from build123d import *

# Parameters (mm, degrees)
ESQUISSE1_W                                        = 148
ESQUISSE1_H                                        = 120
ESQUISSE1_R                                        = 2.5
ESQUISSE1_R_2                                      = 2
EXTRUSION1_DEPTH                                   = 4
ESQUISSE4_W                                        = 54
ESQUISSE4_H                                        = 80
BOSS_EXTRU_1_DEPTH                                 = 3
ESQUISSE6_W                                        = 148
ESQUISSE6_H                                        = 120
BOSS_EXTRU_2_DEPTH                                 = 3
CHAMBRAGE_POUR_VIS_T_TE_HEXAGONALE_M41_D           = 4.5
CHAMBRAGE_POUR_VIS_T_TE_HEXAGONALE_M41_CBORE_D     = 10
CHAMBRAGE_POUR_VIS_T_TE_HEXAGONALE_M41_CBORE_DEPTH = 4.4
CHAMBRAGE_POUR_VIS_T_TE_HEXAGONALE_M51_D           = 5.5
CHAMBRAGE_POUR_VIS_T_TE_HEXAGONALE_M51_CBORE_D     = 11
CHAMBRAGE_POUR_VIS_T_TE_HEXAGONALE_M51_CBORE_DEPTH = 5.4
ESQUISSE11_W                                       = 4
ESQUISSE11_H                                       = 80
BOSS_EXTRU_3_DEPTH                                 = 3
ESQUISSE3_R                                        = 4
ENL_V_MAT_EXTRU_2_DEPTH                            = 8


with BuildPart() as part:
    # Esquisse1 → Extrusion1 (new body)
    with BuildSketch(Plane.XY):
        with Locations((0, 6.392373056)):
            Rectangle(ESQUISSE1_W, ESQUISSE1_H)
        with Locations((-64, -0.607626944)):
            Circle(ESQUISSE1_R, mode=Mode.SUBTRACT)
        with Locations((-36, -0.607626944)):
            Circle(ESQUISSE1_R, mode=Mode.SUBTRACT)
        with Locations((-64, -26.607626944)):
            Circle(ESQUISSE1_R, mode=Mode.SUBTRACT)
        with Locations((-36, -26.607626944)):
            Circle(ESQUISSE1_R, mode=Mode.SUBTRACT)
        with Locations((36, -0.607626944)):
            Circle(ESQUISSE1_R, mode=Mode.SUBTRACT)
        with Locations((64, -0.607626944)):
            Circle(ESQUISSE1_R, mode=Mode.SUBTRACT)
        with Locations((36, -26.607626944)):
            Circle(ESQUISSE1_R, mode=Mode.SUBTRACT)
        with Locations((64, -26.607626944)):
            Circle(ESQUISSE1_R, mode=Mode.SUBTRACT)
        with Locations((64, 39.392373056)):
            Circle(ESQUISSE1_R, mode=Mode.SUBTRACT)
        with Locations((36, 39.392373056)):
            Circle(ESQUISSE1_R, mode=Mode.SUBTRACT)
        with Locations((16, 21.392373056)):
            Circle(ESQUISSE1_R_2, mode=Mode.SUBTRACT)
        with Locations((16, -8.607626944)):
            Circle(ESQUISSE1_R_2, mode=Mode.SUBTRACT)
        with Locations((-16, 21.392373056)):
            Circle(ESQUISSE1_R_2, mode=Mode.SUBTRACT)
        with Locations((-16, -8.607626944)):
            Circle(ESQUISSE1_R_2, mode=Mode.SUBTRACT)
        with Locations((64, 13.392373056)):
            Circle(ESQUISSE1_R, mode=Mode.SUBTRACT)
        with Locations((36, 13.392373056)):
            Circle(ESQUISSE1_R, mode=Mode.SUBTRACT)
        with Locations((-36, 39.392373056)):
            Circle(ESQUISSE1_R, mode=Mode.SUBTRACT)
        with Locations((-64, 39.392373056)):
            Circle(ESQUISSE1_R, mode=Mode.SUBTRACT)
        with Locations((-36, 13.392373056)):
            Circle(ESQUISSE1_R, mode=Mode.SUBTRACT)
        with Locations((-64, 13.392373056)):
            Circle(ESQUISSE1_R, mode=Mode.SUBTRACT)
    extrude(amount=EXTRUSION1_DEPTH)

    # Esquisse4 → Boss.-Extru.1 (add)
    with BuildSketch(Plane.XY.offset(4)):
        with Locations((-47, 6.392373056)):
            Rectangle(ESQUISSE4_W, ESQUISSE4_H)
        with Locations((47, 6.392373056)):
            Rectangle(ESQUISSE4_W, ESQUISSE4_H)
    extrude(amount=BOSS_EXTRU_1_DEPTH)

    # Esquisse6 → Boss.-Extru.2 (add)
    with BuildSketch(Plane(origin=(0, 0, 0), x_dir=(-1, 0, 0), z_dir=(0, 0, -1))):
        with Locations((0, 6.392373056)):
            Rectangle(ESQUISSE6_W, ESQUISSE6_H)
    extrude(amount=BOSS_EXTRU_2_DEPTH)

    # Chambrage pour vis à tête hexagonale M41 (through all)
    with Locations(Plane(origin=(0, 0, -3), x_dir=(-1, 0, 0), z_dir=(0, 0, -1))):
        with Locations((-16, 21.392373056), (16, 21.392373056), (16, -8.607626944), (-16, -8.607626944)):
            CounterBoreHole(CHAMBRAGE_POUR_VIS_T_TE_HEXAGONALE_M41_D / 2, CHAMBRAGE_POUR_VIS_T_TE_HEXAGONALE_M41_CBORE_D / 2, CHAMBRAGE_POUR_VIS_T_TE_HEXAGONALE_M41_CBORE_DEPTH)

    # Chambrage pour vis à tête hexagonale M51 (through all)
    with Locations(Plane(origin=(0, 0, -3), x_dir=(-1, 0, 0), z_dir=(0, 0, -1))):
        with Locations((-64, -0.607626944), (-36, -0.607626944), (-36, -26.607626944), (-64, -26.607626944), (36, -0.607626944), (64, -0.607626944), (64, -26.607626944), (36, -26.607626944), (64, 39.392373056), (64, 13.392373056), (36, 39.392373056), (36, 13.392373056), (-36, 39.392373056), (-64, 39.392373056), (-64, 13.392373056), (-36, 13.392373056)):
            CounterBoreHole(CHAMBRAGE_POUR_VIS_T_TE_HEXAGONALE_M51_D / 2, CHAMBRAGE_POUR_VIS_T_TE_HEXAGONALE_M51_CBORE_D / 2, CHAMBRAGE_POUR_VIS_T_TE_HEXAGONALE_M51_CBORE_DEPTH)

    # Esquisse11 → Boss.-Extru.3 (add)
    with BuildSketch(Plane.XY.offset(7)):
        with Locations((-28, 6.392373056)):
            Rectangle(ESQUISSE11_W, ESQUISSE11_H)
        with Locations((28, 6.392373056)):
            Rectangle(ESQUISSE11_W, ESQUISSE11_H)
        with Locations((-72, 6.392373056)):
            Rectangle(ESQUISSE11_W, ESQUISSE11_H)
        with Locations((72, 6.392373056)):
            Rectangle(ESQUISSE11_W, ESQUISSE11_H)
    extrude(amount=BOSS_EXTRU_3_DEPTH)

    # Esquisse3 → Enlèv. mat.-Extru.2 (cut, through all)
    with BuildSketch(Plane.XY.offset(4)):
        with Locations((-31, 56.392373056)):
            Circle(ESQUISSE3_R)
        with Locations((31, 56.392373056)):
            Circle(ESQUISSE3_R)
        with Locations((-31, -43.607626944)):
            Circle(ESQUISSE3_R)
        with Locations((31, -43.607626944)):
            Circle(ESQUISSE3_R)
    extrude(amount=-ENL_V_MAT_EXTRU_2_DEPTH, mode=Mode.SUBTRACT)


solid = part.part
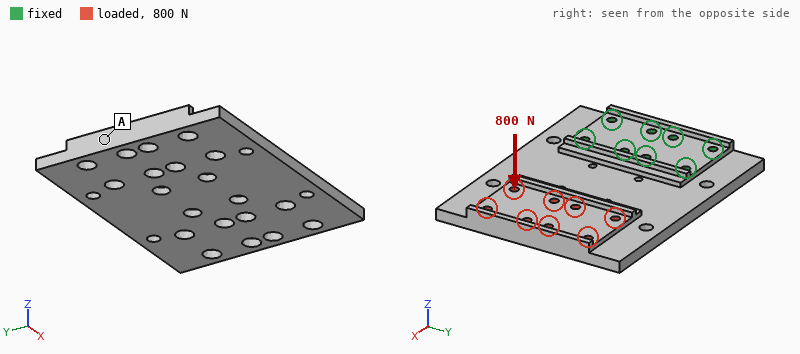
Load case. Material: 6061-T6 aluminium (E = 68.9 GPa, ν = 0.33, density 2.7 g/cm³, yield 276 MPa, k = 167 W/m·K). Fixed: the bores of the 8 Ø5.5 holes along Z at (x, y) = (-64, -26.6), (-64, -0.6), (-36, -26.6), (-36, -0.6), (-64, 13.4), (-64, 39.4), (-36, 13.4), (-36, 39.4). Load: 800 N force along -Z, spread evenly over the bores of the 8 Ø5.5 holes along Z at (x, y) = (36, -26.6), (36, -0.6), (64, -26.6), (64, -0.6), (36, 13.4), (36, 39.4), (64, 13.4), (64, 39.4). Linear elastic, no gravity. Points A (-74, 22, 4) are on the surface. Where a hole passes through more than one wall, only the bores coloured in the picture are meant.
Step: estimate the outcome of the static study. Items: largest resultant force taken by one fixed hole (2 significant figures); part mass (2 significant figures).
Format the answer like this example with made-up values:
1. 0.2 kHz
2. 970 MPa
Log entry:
1. 1.2 kN
2. 380 g
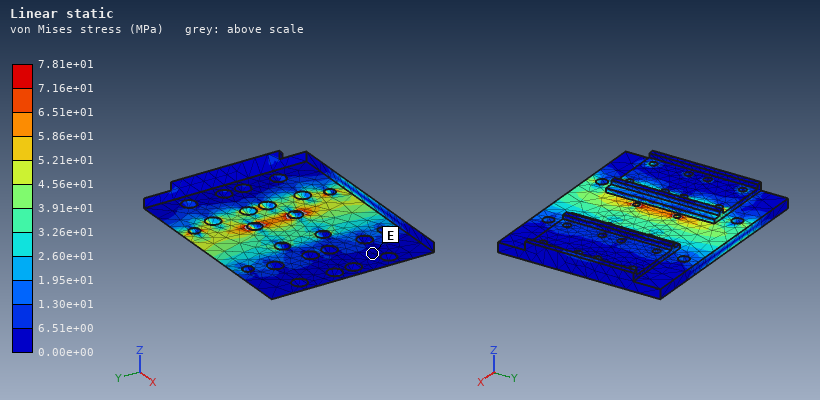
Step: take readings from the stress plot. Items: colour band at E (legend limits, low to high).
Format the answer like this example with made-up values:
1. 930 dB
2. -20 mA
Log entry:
1. 0.00e+00 to 6.51e+00 MPa
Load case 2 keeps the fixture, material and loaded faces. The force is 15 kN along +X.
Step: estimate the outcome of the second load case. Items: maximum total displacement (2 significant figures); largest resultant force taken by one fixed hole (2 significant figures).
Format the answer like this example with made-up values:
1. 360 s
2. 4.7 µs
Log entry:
1. 1.1 mm
2. 4.0 kN
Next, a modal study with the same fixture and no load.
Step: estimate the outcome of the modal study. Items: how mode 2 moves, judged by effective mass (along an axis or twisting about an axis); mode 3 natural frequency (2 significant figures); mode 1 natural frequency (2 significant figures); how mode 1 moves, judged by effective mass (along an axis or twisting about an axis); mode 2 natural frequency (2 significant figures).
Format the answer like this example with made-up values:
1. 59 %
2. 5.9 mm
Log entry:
1. twisting about X
2. 2900 Hz
3. 460 Hz
4. along Z
5. 1100 Hz
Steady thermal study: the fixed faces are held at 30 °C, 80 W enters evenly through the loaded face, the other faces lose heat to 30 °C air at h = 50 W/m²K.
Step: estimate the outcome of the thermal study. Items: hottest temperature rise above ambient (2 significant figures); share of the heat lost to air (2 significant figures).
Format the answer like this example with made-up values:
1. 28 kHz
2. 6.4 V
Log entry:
1. 37 K
2. 44 %
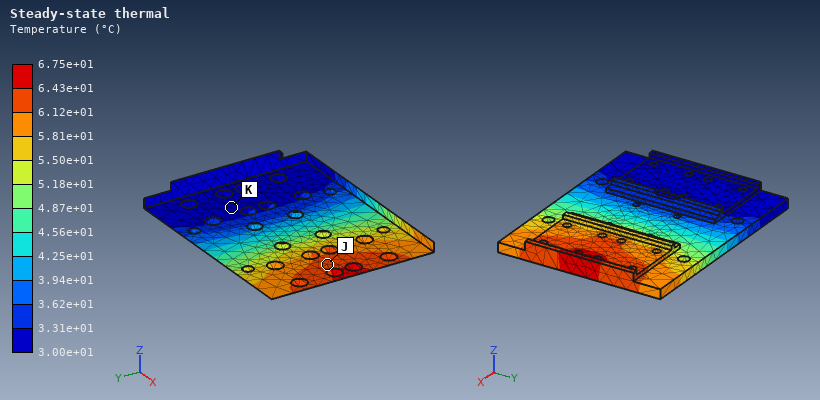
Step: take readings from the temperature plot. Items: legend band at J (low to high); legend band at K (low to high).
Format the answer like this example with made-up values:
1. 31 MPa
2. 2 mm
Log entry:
1. 6.12e+01 to 6.43e+01 °C
2. 3.00e+01 to 3.31e+01 °C
